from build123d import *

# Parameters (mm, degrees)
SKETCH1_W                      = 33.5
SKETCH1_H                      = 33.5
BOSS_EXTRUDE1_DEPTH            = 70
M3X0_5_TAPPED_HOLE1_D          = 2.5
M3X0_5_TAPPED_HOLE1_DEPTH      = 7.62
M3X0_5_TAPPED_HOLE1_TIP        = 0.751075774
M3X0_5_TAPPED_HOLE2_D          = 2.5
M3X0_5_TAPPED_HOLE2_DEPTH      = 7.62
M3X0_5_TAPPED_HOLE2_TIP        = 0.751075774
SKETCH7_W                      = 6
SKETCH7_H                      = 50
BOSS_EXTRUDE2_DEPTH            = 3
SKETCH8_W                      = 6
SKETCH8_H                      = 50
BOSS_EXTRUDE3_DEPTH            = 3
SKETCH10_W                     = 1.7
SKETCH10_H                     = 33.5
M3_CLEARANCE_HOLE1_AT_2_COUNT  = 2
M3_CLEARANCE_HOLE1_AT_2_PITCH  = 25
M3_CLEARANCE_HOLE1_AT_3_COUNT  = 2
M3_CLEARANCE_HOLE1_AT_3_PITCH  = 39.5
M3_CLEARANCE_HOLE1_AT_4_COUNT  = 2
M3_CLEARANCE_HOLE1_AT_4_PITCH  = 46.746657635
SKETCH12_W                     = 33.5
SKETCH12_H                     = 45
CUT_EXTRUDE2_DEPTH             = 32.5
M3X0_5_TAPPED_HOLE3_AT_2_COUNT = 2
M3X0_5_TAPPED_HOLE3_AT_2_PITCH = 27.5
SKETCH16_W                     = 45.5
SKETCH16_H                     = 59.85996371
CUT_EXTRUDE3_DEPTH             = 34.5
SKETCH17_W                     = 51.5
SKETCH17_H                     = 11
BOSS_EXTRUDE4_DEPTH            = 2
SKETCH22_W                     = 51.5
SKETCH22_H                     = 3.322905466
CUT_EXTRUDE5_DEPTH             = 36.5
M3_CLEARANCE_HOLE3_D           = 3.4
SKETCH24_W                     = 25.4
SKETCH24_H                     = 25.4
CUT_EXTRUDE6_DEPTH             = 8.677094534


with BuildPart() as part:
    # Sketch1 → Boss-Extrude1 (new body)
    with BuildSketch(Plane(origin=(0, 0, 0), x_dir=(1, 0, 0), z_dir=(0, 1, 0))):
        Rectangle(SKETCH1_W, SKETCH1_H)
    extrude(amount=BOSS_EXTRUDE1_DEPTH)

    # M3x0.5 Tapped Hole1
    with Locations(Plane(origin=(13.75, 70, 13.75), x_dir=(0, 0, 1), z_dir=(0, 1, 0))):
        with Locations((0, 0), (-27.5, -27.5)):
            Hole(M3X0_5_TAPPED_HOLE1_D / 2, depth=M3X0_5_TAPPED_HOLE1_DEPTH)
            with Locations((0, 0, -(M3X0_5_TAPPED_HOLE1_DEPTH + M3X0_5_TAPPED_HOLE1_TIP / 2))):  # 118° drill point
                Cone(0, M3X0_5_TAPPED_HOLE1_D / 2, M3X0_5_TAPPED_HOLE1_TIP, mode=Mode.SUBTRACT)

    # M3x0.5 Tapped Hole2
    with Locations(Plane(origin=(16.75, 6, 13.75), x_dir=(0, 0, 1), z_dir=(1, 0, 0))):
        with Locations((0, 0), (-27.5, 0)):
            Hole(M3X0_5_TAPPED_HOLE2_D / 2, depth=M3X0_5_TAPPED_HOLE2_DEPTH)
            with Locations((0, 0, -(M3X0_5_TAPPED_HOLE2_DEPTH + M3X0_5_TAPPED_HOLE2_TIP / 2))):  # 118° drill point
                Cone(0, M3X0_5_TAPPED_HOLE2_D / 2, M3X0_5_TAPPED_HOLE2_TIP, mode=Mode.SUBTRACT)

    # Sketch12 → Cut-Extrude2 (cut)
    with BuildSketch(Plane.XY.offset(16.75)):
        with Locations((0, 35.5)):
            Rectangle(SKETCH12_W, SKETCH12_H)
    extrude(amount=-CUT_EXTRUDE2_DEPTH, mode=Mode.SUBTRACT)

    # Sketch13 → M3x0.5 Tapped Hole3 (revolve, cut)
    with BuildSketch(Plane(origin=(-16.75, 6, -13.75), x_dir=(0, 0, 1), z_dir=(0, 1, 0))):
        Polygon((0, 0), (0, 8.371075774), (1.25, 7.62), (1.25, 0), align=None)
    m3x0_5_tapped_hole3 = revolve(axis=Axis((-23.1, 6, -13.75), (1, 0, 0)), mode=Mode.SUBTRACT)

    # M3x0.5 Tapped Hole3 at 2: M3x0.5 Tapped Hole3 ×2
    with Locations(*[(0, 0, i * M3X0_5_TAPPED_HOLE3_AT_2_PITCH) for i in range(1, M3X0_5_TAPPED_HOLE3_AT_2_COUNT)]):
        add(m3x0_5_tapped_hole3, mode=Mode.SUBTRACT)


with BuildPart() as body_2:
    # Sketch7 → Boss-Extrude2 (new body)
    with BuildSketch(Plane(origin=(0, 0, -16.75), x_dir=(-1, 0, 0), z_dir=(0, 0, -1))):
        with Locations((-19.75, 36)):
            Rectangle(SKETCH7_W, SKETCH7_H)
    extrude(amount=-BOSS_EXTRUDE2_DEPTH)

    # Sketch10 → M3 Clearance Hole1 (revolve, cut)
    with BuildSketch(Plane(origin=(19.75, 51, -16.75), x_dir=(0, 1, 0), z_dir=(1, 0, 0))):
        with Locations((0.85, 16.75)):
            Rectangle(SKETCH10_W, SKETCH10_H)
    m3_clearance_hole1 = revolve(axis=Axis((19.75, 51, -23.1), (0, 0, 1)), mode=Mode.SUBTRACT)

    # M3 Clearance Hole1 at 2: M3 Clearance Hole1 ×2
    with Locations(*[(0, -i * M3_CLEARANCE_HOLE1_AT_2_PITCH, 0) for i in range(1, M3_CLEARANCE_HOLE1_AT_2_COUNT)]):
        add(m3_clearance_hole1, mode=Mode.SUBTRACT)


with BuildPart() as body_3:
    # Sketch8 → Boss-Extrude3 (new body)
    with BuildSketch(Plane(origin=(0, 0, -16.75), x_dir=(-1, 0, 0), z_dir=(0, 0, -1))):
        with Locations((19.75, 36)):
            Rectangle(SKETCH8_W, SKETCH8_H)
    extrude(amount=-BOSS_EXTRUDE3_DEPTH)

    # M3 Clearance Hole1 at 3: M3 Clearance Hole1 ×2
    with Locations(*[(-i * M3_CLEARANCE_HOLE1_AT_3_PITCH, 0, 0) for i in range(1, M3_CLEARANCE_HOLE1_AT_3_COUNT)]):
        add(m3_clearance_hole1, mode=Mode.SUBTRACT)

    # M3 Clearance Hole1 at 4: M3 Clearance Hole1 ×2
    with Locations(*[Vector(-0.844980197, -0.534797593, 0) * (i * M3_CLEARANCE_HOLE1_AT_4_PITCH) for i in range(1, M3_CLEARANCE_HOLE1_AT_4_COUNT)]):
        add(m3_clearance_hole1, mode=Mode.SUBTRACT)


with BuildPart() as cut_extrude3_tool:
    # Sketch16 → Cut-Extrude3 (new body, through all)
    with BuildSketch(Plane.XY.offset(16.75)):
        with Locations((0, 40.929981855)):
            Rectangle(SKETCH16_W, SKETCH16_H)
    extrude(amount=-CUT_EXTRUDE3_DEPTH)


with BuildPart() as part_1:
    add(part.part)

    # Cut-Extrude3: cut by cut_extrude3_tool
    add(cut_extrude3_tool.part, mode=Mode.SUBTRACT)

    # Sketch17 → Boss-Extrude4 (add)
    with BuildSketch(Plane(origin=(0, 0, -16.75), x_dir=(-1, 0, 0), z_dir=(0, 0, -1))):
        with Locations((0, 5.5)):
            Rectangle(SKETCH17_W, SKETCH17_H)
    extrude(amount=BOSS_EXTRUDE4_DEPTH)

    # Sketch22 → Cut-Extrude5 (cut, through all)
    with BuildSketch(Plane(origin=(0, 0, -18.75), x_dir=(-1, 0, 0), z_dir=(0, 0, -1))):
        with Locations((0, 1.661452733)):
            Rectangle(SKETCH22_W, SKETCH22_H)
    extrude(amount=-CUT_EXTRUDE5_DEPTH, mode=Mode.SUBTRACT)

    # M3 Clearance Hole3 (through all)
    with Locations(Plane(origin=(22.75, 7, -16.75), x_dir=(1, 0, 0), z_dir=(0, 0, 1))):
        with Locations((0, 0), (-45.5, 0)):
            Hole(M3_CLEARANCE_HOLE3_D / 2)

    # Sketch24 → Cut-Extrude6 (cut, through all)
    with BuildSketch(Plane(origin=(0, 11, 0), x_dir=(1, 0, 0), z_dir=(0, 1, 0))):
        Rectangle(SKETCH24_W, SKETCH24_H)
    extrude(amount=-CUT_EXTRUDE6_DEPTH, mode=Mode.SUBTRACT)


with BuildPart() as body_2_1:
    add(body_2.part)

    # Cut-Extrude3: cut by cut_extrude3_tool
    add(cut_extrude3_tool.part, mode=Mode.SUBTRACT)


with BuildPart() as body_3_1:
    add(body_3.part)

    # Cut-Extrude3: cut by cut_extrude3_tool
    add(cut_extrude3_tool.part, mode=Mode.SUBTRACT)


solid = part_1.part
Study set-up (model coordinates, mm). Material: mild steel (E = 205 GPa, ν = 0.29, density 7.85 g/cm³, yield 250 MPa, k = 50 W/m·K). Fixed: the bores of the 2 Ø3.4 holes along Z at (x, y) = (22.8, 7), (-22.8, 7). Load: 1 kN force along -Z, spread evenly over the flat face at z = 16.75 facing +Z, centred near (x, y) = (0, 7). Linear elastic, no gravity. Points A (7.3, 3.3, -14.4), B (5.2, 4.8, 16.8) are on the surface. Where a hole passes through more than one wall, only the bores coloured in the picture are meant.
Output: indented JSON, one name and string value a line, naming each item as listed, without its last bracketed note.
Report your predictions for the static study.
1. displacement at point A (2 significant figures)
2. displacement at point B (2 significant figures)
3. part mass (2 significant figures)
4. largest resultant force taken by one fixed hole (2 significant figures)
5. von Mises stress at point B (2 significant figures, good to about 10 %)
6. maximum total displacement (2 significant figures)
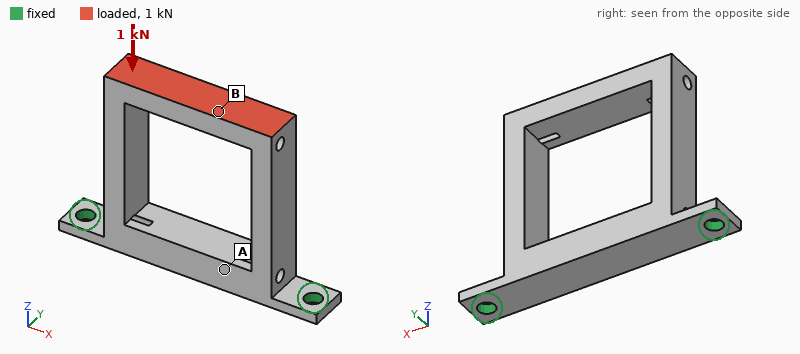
{
  "displacement at point A": "13 µm",
  "displacement at point B": "28 µm",
  "part mass": "33 g",
  "largest resultant force taken by one fixed hole": "560 N",
  "von Mises stress at point B": "63 MPa",
  "maximum total displacement": "31 µm"
}
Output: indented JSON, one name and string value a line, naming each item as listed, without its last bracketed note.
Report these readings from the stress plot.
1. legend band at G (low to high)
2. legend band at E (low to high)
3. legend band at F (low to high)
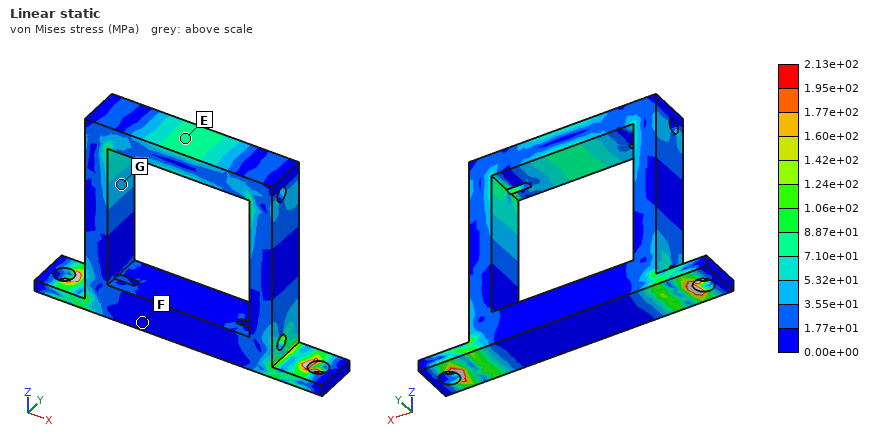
{
  "legend band at G": "3.55e+01 to 5.32e+01 MPa",
  "legend band at E": "7.10e+01 to 8.87e+01 MPa",
  "legend band at F": "0.00e+00 to 1.77e+01 MPa"
}
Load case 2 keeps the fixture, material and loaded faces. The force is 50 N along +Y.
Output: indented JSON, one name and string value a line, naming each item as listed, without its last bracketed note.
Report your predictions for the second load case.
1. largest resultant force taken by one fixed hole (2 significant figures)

{
  "largest resultant force taken by one fixed hole": "25 N"
}
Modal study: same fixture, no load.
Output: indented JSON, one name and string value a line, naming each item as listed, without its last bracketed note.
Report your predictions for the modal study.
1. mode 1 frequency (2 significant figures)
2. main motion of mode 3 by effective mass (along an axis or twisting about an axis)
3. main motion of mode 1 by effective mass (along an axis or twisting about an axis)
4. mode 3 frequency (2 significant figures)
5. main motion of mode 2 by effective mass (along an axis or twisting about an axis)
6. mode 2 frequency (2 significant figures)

{
  "mode 1 frequency": "1100 Hz",
  "main motion of mode 3 by effective mass": "twisting about Z",
  "main motion of mode 1 by effective mass": "along Y",
  "mode 3 frequency": "4700 Hz",
  "main motion of mode 2 by effective mass": "along X",
  "mode 2 frequency": "3000 Hz"
}
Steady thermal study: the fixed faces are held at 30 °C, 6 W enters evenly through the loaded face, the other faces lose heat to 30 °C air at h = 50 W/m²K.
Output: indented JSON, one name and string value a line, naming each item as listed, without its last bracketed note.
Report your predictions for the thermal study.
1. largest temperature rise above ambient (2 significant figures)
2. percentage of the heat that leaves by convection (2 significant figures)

{
  "largest temperature rise above ambient": "55 K",
  "percentage of the heat that leaves by convection": "62 %"
}
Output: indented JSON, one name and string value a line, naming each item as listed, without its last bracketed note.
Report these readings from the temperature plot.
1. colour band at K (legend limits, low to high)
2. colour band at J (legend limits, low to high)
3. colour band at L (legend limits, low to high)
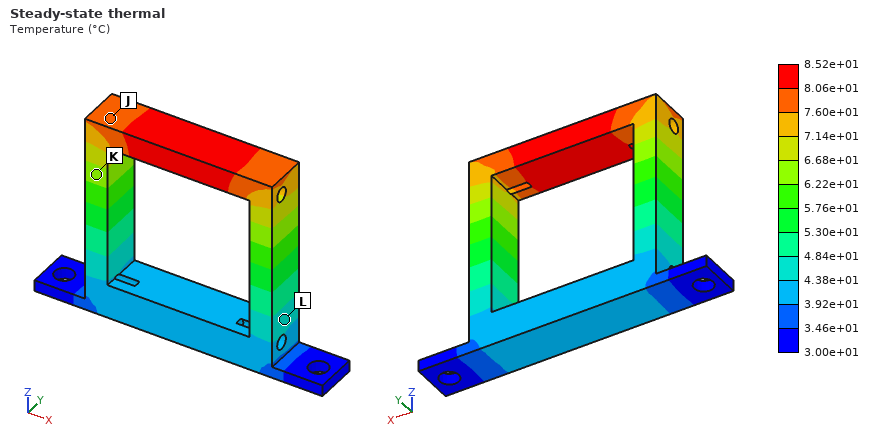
{
  "colour band at K": "6.22e+01 to 6.68e+01 °C",
  "colour band at J": "7.60e+01 to 8.06e+01 °C",
  "colour band at L": "4.38e+01 to 4.84e+01 °C"
}
